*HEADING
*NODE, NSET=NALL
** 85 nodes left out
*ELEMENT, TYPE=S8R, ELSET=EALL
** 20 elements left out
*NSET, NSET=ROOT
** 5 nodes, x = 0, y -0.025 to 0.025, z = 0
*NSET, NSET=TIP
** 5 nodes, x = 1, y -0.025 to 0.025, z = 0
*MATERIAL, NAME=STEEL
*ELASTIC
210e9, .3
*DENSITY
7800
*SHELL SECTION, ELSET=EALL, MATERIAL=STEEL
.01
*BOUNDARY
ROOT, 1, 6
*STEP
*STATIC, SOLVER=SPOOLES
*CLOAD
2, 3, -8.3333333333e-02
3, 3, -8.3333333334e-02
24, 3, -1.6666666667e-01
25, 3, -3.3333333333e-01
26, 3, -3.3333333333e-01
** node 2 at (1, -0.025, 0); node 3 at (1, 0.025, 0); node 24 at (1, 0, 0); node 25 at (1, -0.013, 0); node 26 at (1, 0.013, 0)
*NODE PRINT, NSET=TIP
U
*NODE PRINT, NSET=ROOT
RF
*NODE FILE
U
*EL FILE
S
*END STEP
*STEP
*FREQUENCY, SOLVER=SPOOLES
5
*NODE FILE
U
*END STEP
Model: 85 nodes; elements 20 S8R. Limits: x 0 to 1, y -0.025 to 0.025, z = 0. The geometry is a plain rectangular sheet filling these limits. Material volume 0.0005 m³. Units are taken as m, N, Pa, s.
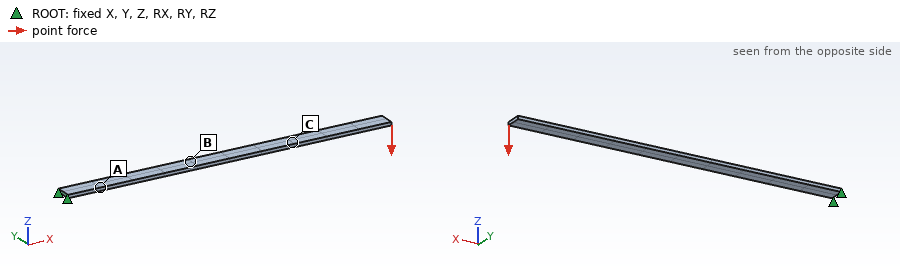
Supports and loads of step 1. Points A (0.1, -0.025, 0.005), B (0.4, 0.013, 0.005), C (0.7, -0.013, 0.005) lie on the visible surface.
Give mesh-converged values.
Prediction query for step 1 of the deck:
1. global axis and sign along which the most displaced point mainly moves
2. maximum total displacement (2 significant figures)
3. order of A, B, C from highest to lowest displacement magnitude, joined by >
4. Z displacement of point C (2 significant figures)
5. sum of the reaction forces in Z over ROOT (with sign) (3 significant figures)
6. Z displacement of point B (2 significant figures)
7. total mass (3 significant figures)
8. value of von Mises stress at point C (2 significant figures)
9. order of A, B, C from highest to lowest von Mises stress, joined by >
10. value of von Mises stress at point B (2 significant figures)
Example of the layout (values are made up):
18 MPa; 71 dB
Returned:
-Z; 3.8e-04 m; C > B > A; -2.1e-04 m; 1.00 N; -7.8e-05 m; 3.90 kg; 3.6e+05 Pa; A > B > C; 7.2e+05 Pa
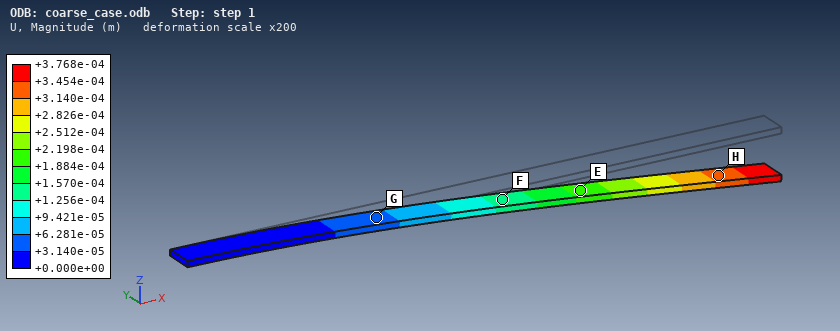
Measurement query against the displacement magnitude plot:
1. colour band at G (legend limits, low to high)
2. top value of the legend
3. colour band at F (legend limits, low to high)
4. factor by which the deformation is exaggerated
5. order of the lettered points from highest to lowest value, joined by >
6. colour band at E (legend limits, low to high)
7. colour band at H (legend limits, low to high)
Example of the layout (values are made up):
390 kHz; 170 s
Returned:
+3.140e-05 to +6.281e-05 m; +3.768e-04 m; +1.256e-04 to +1.570e-04 m; 200; H > E > F > G; +1.884e-04 to +2.198e-04 m; +3.140e-04 to +3.454e-04 m
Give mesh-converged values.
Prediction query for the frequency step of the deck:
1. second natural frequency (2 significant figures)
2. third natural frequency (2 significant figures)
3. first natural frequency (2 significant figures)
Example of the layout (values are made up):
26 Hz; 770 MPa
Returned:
42 Hz; 53 Hz; 8.4 Hz
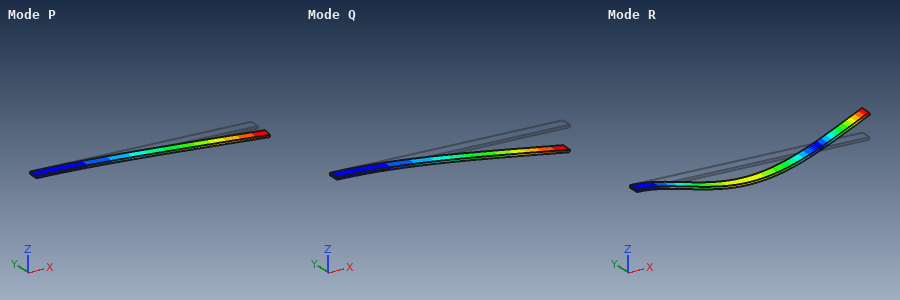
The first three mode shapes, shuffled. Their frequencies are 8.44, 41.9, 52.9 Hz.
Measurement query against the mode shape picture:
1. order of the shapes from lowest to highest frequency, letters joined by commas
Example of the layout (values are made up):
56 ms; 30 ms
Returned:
Q, P, R
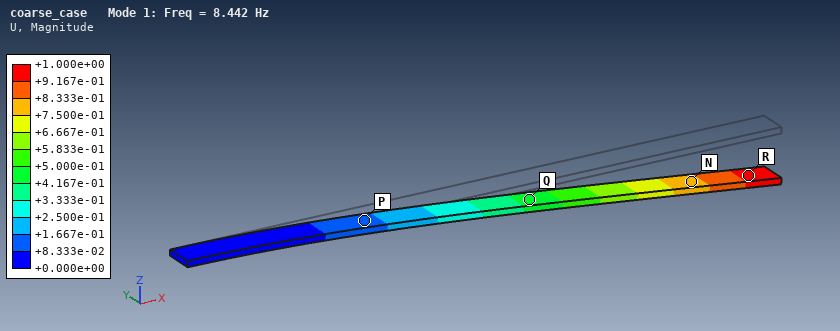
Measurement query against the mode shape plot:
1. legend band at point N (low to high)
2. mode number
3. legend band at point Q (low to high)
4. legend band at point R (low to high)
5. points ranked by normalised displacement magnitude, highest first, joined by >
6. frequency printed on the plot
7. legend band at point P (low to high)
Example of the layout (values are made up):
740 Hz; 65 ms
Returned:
+7.500e-01 to +8.333e-01; 1; +4.167e-01 to +5.000e-01; +9.167e-01 to +1.000e+00; R > N > Q > P; 8.442 Hz; +8.333e-02 to +1.667e-01
